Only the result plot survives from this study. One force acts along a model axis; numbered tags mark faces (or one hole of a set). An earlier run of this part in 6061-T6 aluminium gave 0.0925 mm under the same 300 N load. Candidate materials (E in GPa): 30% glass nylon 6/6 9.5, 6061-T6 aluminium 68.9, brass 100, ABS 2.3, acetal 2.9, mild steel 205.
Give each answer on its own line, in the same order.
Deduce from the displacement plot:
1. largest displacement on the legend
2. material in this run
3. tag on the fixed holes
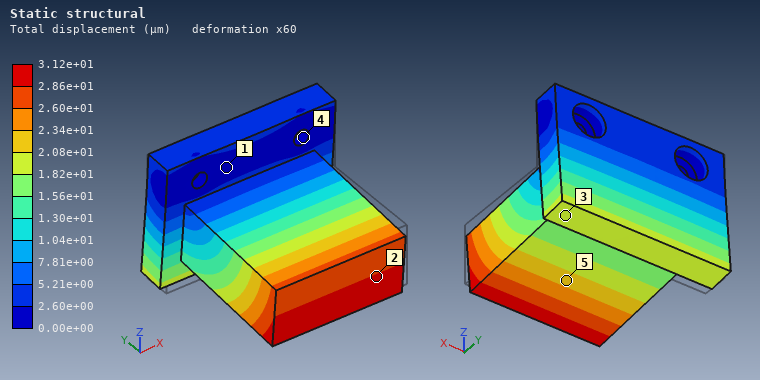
3.12e+01 µm
mild steel
4
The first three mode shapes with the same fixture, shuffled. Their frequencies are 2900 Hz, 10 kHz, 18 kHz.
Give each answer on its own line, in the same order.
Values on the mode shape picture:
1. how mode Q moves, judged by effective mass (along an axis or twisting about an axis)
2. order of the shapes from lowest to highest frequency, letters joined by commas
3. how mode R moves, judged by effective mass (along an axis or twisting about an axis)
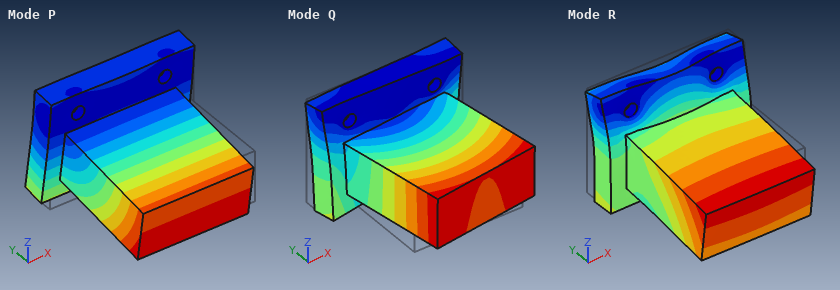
along X
P, Q, R
along Y
